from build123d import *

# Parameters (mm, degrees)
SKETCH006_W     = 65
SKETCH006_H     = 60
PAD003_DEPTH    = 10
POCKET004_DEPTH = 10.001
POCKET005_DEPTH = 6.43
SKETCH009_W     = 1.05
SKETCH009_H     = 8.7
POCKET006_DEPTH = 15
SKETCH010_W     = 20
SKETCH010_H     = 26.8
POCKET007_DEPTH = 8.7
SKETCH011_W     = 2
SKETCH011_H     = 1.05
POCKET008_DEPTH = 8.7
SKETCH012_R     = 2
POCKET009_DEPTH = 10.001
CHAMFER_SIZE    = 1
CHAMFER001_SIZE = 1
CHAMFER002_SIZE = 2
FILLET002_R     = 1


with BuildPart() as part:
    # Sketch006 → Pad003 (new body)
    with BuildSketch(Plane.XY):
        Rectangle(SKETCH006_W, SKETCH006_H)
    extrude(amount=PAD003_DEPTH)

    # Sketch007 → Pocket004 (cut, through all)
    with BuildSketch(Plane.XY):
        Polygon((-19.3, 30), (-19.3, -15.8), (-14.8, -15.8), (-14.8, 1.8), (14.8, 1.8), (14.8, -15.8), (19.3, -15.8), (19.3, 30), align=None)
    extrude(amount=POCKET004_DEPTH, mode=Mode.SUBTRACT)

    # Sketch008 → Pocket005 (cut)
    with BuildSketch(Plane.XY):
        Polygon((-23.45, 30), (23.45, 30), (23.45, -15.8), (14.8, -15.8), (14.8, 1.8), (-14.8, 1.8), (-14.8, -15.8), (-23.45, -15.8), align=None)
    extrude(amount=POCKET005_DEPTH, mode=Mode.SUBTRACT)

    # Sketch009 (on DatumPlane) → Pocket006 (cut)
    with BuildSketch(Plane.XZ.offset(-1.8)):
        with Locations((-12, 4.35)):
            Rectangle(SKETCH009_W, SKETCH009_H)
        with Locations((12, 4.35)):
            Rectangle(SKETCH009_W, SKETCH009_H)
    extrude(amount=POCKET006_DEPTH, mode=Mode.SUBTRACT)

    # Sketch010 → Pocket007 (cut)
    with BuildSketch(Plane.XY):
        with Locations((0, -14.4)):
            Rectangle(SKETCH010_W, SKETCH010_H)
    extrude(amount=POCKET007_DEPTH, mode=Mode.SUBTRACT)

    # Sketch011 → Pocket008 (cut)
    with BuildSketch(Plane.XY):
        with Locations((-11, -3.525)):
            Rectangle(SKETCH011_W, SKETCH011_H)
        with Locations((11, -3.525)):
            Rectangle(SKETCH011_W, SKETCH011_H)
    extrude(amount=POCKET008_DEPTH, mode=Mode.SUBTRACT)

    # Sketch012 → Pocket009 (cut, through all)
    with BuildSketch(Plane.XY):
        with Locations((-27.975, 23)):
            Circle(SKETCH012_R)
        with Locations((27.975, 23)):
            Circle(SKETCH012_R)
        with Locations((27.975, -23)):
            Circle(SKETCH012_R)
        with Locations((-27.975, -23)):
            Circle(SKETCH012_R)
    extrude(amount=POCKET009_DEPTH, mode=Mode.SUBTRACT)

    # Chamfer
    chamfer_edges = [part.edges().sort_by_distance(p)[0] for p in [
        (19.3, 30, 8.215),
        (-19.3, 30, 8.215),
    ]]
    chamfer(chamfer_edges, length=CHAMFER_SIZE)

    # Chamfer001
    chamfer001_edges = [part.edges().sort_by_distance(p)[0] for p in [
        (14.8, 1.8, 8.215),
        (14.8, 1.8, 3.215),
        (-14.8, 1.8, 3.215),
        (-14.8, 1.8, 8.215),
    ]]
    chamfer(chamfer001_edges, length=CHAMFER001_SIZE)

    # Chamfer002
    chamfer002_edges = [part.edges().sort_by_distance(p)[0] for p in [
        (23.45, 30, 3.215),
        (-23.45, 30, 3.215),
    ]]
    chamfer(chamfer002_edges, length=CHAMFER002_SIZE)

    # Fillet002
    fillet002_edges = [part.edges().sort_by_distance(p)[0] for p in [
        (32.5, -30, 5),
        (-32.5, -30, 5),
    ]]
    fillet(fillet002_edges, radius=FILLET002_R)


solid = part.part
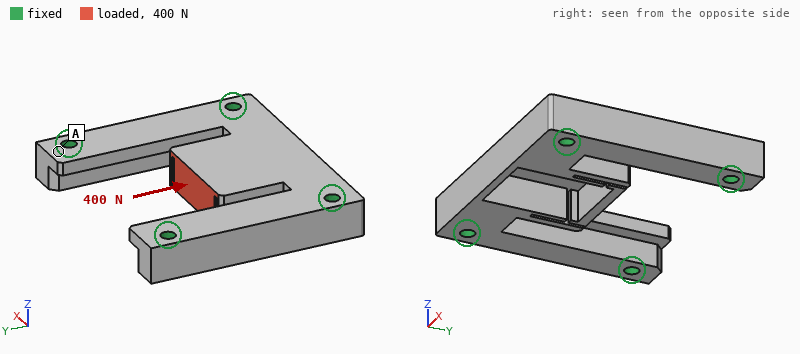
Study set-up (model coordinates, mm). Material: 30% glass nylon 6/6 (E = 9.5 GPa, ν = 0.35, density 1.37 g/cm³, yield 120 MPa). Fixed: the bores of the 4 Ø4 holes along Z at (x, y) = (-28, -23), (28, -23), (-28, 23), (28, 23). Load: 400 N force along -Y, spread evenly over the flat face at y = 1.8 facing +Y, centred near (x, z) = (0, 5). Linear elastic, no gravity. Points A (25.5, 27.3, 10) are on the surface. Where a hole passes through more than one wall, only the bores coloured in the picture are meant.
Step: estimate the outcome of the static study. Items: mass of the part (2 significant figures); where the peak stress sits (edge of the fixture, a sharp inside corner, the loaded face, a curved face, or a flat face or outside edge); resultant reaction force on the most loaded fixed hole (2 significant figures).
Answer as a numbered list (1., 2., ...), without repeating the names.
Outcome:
1. 25 g
2. the loaded face
3. 160 N
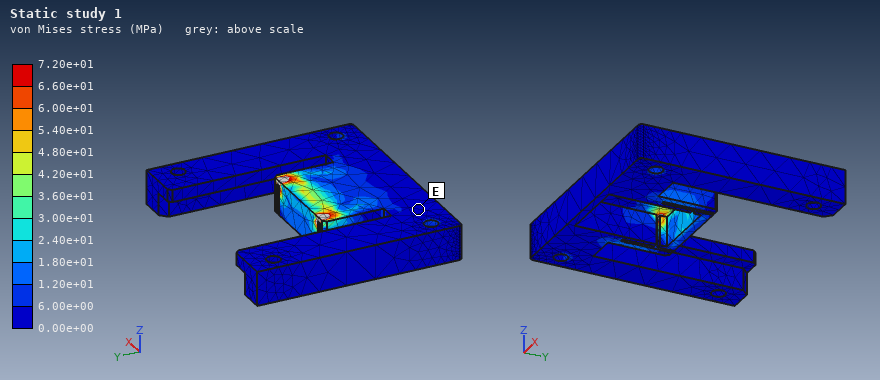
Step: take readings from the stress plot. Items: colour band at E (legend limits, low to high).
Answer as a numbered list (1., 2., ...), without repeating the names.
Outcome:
1. 0.00e+00 to 6.00e+00 MPa
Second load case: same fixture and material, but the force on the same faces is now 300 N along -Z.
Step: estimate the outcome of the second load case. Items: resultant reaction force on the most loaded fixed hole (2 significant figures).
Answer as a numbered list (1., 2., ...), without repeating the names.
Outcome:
1. 140 N
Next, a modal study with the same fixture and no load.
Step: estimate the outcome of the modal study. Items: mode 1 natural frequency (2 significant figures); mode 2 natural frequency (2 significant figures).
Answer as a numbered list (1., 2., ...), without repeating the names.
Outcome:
1. 3600 Hz
2. 4500 Hz
